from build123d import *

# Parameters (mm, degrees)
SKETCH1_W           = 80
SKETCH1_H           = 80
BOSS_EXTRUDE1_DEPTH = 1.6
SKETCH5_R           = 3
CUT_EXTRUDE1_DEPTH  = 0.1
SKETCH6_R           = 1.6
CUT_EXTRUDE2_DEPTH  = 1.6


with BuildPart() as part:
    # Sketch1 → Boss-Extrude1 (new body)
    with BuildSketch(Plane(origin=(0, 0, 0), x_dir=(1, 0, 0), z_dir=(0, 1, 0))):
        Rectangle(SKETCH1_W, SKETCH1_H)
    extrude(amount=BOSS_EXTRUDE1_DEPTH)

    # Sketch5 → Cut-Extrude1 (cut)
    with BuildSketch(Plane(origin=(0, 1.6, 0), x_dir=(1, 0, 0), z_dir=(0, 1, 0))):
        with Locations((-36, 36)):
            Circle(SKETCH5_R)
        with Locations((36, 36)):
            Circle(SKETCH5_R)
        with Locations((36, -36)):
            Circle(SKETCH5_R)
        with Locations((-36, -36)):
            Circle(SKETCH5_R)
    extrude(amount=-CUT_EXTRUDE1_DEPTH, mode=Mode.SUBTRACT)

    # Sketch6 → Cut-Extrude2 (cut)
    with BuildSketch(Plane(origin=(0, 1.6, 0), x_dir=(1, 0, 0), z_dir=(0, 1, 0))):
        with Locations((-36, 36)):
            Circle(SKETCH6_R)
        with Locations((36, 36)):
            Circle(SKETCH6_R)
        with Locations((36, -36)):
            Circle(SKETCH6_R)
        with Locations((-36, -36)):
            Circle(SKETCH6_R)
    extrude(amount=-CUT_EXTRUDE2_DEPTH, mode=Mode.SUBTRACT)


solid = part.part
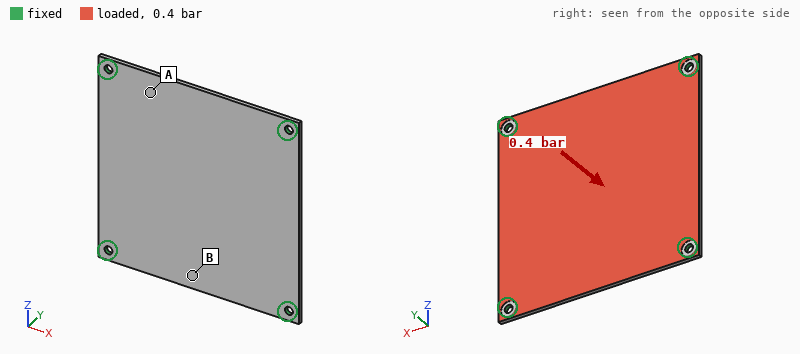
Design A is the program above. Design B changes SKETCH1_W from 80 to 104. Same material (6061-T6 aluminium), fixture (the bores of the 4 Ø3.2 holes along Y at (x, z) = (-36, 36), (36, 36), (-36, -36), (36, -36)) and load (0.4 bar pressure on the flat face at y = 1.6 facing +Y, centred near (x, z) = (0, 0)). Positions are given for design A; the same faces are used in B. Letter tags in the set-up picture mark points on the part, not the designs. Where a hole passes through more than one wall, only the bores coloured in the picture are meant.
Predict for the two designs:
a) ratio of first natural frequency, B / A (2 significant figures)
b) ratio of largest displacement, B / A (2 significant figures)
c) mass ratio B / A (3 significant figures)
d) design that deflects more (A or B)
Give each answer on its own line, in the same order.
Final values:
1.1
0.91
1.30
A
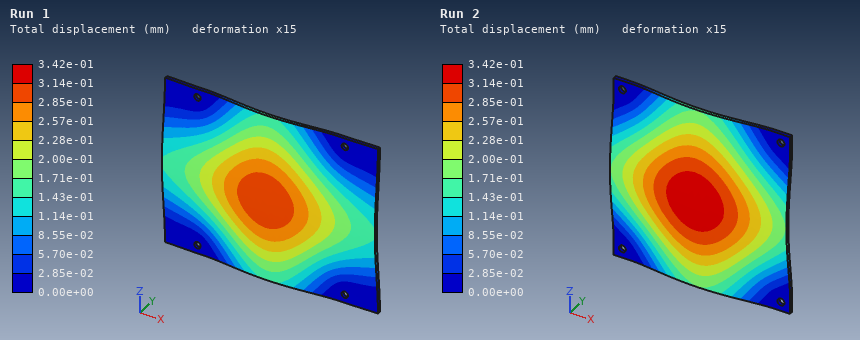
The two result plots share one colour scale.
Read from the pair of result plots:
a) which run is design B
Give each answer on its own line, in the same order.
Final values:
Run 1
